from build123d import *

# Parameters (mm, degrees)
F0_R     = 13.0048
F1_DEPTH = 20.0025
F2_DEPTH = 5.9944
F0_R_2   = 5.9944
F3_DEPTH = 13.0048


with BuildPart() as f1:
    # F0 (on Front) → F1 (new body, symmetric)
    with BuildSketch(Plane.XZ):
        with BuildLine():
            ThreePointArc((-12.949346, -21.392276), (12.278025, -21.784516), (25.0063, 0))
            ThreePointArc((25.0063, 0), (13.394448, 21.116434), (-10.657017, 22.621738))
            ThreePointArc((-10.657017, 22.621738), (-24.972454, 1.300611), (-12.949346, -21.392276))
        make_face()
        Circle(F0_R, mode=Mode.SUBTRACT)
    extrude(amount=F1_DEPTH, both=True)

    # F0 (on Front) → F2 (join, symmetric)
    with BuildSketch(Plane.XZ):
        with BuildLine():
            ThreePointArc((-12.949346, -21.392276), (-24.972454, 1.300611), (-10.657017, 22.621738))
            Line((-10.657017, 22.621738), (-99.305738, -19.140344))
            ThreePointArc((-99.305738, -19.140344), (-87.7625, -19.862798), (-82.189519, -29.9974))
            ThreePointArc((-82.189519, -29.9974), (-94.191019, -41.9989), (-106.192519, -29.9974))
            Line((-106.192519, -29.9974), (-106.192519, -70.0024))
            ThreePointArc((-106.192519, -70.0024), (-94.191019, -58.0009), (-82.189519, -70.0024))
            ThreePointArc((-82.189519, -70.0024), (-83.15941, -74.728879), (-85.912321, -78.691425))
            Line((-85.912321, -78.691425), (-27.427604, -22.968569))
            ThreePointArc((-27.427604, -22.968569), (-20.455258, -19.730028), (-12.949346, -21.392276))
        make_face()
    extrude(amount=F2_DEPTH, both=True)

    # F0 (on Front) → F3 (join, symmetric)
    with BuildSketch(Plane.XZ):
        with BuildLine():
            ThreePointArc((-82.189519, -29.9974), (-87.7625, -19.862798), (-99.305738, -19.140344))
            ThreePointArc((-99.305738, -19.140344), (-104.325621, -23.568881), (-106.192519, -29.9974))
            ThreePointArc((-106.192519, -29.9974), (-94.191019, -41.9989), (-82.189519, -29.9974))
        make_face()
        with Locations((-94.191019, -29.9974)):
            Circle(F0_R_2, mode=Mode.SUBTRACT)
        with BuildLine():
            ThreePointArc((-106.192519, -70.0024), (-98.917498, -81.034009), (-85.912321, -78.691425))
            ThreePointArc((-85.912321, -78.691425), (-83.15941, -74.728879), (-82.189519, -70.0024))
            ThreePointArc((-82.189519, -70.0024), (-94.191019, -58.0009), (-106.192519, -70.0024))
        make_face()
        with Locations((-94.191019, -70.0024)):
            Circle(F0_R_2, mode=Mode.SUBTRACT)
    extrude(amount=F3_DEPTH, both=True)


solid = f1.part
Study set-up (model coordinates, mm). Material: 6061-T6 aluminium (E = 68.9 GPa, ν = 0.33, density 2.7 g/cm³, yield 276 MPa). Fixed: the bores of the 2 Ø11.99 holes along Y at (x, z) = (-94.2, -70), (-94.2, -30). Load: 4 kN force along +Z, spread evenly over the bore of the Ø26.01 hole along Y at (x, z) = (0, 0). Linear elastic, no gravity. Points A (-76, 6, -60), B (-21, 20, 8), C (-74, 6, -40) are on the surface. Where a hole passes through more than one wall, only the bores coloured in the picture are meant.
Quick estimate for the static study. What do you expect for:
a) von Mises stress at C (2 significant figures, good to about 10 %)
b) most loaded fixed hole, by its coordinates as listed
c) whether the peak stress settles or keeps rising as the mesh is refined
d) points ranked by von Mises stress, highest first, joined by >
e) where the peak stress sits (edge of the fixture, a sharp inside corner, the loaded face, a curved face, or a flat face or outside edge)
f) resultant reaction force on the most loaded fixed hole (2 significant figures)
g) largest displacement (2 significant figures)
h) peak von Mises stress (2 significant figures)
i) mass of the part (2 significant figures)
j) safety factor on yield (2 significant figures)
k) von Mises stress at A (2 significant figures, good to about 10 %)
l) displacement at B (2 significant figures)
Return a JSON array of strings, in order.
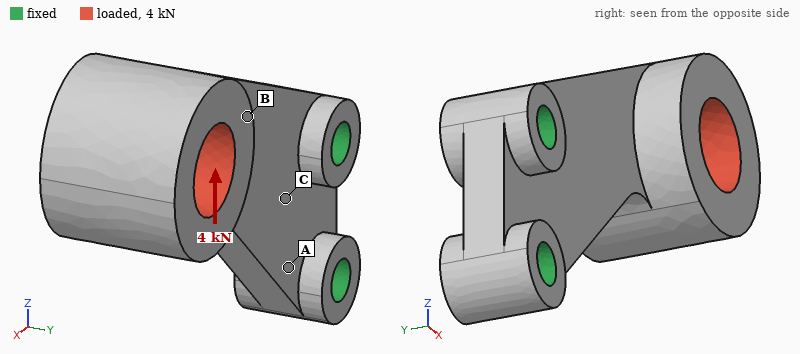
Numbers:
["21 MPa", "(-94.2, -70)", "settles", "A > C > B", "a curved face", "9.2 kN", "0.33 mm", "91 MPa", "320 g", "3.0", "44 MPa", "0.17 mm"]
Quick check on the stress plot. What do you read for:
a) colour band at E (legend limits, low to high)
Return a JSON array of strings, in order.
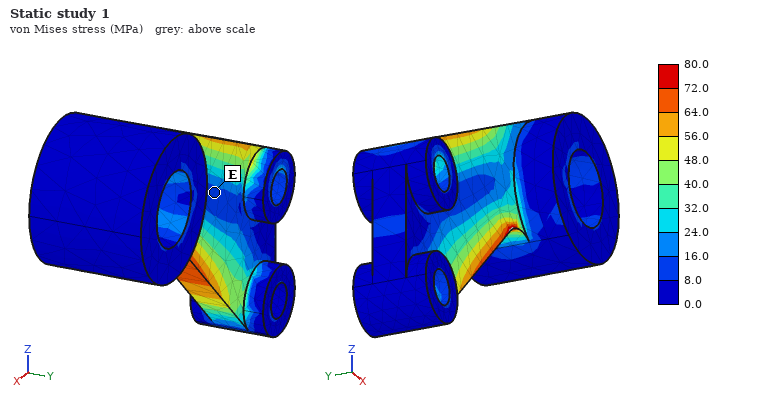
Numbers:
["8.0 to 16.0 MPa"]
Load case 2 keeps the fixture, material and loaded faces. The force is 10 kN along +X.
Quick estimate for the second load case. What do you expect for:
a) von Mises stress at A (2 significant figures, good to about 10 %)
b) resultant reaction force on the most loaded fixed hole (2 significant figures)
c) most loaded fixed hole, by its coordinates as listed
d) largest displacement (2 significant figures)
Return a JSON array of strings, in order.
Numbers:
["35 MPa", "16 kN", "(-94.2, -30)", "0.29 mm"]
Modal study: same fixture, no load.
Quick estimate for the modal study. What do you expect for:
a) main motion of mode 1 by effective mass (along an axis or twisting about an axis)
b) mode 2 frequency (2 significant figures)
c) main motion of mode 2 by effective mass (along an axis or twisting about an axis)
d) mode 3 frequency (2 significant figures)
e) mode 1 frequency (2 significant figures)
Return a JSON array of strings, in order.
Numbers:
["along Y", "1500 Hz", "along Z", "1800 Hz", "480 Hz"]
